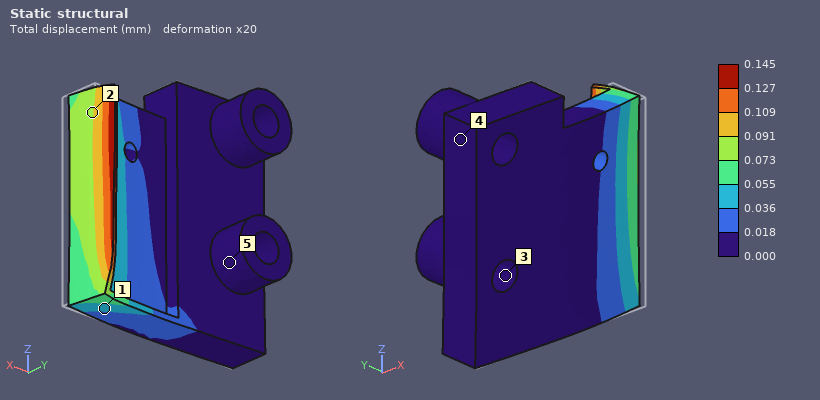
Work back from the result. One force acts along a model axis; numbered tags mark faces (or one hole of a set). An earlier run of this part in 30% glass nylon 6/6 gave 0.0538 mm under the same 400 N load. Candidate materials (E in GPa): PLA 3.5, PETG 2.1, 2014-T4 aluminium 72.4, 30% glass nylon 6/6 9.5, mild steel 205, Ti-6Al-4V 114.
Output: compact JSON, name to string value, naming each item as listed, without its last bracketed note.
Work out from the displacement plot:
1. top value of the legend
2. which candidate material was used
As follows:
{"top value of the legend": "0.145 mm", "which candidate material was used": "PLA"}
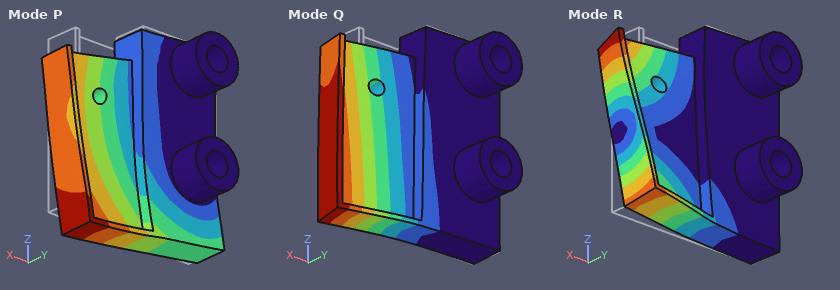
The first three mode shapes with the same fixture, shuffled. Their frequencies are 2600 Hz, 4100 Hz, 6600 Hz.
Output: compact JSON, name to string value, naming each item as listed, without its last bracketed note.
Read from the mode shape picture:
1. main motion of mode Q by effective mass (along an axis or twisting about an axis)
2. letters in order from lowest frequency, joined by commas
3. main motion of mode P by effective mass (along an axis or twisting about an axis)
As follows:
{"main motion of mode Q by effective mass": "along Y", "letters in order from lowest frequency, joined by commas": "Q, R, P", "main motion of mode P by effective mass": "along Z"}
